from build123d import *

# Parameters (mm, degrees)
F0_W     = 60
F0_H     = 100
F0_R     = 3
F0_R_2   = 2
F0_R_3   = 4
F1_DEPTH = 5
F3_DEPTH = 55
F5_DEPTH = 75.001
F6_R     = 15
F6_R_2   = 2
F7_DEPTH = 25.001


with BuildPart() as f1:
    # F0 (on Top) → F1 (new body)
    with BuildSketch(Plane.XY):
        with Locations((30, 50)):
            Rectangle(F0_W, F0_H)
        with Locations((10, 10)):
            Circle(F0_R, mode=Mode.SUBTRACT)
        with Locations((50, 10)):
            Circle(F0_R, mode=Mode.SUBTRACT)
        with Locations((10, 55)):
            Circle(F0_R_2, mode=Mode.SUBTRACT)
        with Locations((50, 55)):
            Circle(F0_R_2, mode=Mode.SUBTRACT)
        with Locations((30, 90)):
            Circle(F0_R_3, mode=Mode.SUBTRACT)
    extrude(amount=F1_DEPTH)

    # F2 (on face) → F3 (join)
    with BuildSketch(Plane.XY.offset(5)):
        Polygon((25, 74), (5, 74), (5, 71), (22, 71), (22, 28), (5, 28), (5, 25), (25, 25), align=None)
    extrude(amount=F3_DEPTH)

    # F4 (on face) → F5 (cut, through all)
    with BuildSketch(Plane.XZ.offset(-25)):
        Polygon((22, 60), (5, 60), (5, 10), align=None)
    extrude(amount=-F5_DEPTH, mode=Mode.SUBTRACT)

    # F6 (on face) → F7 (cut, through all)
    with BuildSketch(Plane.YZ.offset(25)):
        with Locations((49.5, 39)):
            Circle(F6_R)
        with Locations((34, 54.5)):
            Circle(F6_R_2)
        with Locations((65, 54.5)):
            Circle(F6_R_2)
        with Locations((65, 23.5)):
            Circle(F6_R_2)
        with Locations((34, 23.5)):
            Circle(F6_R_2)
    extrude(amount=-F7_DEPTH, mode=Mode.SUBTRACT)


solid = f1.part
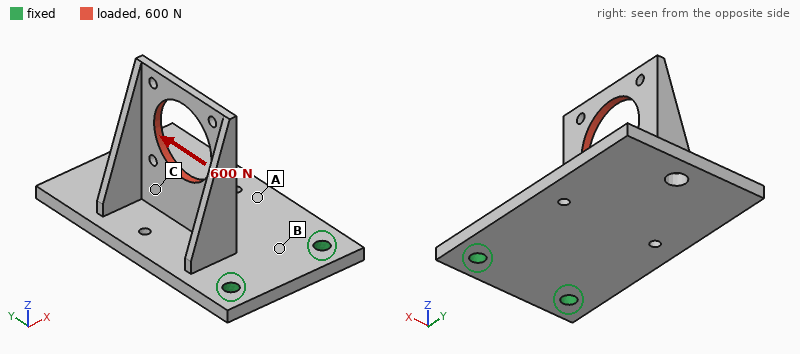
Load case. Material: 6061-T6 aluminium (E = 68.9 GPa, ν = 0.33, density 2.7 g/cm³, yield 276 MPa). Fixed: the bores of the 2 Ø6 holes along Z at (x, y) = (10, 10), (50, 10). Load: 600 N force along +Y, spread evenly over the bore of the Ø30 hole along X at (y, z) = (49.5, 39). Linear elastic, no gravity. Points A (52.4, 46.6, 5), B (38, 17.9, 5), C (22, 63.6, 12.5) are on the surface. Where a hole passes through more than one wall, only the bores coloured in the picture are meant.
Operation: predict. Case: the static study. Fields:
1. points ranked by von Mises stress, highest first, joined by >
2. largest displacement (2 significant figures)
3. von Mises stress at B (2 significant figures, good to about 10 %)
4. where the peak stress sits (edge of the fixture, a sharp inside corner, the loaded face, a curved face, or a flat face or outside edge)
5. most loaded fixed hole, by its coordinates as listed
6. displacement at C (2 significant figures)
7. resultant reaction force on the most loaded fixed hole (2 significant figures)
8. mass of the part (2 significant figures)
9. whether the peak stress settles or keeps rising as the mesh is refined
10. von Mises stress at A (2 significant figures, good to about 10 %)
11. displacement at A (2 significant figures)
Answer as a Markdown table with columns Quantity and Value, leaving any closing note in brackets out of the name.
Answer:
| Quantity | Value |
|---|---|
| points ranked by von Mises stress, highest first, joined by > | B > A > C |
| largest displacement | 1.00 mm |
| von Mises stress at B | 66 MPa |
| where the peak stress sits | edge of the fixture |
| most loaded fixed hole, by its coordinates as listed | (10, 10) |
| displacement at C | 0.52 mm |
| resultant reaction force on the most loaded fixed hole | 420 N |
| mass of the part | 100 g |
| whether the peak stress settles or keeps rising as the mesh is refined | keeps rising |
| von Mises stress at A | 20 MPa |
| displacement at A | 0.24 mm |
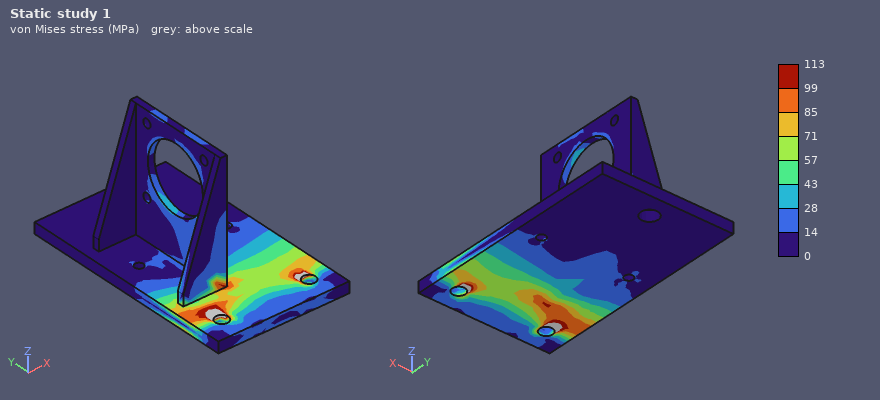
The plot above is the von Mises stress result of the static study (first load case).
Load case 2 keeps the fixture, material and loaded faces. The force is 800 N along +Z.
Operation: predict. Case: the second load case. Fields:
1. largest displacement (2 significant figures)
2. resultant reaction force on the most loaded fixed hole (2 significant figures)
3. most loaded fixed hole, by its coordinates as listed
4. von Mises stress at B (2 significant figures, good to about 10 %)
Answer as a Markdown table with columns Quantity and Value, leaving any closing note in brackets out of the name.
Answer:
| Quantity | Value |
|---|---|
| largest displacement | 1.1 mm |
| resultant reaction force on the most loaded fixed hole | 500 N |
| most loaded fixed hole, by its coordinates as listed | (10, 10) |
| von Mises stress at B | 74 MPa |
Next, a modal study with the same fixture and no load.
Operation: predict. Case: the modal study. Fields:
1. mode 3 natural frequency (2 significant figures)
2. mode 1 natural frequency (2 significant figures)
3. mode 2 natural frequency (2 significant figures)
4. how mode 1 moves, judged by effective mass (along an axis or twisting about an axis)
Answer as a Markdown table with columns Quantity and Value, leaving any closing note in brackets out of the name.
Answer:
| Quantity | Value |
|---|---|
| mode 3 natural frequency | 3000 Hz |
| mode 1 natural frequency | 500 Hz |
| mode 2 natural frequency | 1300 Hz |
| how mode 1 moves, judged by effective mass | along Z |
